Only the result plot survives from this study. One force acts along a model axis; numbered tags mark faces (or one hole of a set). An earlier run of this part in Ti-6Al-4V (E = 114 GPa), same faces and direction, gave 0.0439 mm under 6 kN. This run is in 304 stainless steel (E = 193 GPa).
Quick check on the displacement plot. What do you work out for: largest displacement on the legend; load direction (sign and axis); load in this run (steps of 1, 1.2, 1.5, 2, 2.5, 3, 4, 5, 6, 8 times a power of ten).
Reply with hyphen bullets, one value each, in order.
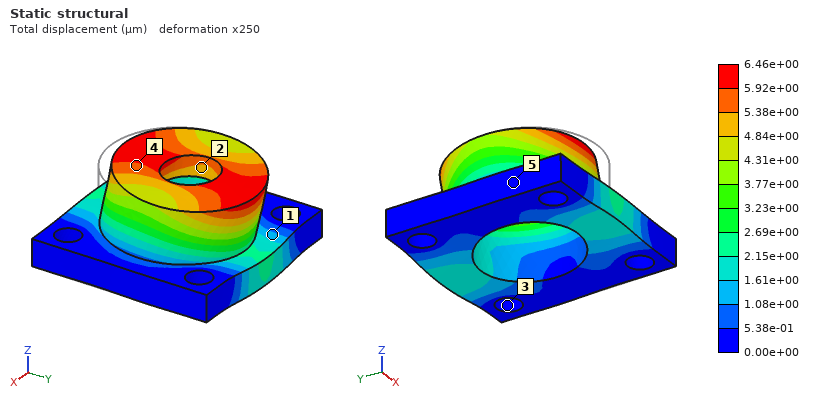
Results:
- 6.46e+00 µm
- +Y
- 1.5 kN
